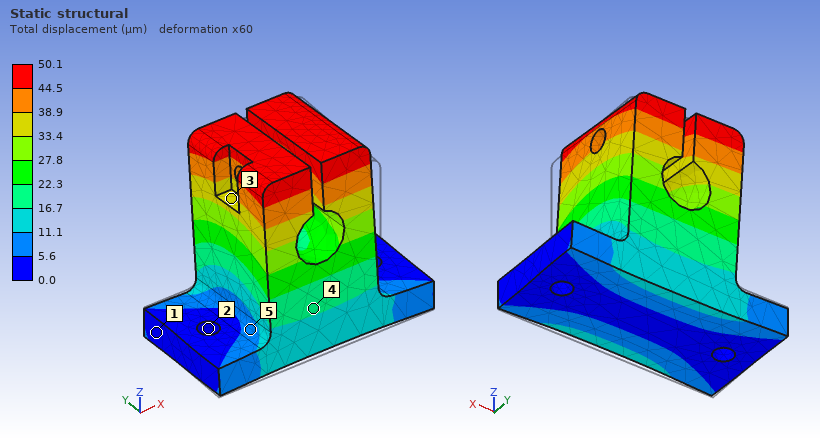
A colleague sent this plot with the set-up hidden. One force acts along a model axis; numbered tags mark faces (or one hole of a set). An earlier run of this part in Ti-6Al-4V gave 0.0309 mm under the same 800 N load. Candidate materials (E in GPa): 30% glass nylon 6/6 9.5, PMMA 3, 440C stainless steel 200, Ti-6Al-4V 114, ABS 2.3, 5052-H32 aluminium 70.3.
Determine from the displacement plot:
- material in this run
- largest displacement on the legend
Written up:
5052-H32 aluminium
50.1 µm
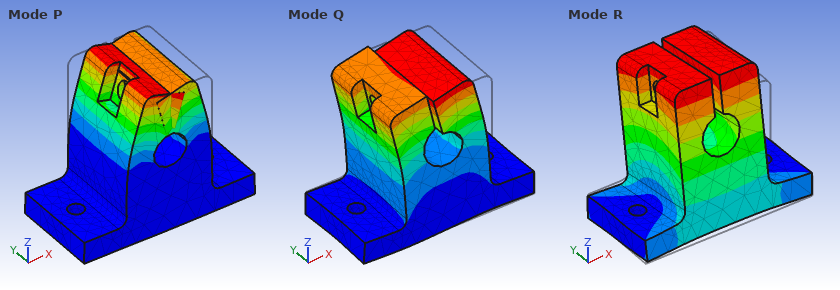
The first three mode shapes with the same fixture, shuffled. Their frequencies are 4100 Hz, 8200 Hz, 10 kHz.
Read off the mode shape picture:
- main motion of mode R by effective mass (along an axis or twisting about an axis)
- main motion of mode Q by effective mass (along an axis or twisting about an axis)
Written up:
along Y
along X
